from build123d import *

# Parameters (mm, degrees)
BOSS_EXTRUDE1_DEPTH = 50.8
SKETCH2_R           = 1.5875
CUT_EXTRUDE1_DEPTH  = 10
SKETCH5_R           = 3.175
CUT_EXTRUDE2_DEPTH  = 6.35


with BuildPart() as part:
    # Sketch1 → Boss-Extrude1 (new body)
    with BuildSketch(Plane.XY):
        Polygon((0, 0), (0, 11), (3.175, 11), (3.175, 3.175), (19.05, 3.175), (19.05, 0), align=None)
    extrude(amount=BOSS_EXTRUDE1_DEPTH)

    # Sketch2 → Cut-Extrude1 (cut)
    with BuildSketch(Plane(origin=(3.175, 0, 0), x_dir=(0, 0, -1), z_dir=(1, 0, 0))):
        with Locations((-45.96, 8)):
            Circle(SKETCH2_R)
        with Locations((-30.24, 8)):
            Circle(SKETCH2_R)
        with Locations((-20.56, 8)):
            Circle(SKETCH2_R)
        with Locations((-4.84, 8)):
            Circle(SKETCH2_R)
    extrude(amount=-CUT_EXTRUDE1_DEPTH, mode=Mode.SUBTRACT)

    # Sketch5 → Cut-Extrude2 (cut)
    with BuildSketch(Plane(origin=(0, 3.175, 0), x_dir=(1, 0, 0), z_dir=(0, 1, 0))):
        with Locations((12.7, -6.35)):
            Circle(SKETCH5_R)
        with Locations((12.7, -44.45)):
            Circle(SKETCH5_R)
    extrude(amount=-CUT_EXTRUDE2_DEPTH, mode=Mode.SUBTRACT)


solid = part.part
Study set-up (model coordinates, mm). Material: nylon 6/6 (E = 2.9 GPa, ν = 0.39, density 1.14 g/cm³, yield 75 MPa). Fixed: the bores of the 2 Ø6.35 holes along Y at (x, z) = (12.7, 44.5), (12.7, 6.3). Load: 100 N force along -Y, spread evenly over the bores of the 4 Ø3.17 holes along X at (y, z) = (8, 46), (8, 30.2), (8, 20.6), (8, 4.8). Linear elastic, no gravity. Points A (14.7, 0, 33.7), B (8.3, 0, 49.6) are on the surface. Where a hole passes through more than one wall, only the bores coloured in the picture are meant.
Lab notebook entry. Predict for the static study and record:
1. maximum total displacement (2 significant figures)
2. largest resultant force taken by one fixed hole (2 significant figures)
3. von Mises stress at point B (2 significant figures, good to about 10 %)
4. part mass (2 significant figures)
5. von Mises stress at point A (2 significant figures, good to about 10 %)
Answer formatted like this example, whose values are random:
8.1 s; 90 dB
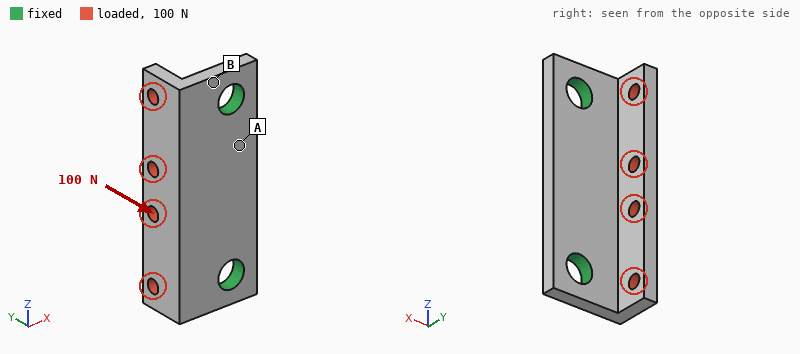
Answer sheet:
0.19 mm; 51 N; 8.5 MPa; 4.6 g; 2.6 MPa
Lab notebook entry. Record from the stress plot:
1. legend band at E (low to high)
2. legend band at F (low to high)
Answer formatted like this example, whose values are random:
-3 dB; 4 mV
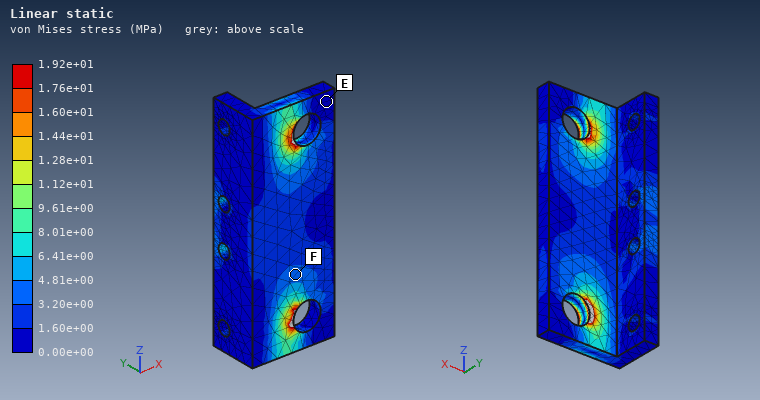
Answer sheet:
0.00e+00 to 1.60e+00 MPa; 3.20e+00 to 4.81e+00 MPa
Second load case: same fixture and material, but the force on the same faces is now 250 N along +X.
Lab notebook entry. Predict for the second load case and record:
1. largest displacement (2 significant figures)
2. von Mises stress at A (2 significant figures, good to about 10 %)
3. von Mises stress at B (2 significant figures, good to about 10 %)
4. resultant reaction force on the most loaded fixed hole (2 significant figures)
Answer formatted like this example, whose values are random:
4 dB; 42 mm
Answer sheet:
0.57 mm; 5.1 MPa; 18 MPa; 130 N
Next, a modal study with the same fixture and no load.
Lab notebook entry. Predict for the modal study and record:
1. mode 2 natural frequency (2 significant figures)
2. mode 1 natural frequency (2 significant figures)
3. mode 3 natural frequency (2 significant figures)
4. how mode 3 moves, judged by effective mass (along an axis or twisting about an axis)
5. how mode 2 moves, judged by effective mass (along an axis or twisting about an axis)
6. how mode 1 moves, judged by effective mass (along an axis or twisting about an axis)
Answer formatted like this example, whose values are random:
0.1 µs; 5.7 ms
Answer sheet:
4100 Hz; 2700 Hz; 4900 Hz; along Y; twisting about X; along Y
